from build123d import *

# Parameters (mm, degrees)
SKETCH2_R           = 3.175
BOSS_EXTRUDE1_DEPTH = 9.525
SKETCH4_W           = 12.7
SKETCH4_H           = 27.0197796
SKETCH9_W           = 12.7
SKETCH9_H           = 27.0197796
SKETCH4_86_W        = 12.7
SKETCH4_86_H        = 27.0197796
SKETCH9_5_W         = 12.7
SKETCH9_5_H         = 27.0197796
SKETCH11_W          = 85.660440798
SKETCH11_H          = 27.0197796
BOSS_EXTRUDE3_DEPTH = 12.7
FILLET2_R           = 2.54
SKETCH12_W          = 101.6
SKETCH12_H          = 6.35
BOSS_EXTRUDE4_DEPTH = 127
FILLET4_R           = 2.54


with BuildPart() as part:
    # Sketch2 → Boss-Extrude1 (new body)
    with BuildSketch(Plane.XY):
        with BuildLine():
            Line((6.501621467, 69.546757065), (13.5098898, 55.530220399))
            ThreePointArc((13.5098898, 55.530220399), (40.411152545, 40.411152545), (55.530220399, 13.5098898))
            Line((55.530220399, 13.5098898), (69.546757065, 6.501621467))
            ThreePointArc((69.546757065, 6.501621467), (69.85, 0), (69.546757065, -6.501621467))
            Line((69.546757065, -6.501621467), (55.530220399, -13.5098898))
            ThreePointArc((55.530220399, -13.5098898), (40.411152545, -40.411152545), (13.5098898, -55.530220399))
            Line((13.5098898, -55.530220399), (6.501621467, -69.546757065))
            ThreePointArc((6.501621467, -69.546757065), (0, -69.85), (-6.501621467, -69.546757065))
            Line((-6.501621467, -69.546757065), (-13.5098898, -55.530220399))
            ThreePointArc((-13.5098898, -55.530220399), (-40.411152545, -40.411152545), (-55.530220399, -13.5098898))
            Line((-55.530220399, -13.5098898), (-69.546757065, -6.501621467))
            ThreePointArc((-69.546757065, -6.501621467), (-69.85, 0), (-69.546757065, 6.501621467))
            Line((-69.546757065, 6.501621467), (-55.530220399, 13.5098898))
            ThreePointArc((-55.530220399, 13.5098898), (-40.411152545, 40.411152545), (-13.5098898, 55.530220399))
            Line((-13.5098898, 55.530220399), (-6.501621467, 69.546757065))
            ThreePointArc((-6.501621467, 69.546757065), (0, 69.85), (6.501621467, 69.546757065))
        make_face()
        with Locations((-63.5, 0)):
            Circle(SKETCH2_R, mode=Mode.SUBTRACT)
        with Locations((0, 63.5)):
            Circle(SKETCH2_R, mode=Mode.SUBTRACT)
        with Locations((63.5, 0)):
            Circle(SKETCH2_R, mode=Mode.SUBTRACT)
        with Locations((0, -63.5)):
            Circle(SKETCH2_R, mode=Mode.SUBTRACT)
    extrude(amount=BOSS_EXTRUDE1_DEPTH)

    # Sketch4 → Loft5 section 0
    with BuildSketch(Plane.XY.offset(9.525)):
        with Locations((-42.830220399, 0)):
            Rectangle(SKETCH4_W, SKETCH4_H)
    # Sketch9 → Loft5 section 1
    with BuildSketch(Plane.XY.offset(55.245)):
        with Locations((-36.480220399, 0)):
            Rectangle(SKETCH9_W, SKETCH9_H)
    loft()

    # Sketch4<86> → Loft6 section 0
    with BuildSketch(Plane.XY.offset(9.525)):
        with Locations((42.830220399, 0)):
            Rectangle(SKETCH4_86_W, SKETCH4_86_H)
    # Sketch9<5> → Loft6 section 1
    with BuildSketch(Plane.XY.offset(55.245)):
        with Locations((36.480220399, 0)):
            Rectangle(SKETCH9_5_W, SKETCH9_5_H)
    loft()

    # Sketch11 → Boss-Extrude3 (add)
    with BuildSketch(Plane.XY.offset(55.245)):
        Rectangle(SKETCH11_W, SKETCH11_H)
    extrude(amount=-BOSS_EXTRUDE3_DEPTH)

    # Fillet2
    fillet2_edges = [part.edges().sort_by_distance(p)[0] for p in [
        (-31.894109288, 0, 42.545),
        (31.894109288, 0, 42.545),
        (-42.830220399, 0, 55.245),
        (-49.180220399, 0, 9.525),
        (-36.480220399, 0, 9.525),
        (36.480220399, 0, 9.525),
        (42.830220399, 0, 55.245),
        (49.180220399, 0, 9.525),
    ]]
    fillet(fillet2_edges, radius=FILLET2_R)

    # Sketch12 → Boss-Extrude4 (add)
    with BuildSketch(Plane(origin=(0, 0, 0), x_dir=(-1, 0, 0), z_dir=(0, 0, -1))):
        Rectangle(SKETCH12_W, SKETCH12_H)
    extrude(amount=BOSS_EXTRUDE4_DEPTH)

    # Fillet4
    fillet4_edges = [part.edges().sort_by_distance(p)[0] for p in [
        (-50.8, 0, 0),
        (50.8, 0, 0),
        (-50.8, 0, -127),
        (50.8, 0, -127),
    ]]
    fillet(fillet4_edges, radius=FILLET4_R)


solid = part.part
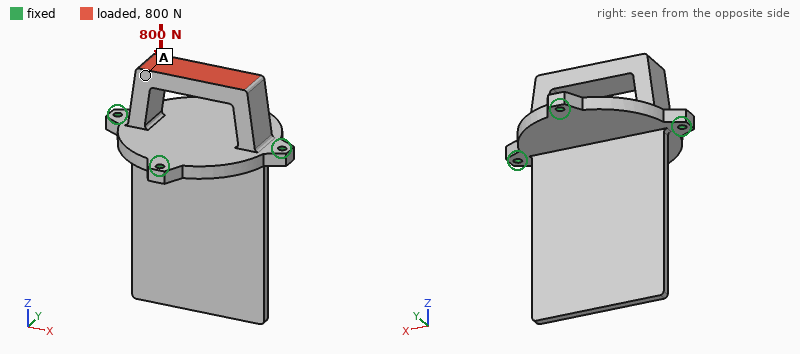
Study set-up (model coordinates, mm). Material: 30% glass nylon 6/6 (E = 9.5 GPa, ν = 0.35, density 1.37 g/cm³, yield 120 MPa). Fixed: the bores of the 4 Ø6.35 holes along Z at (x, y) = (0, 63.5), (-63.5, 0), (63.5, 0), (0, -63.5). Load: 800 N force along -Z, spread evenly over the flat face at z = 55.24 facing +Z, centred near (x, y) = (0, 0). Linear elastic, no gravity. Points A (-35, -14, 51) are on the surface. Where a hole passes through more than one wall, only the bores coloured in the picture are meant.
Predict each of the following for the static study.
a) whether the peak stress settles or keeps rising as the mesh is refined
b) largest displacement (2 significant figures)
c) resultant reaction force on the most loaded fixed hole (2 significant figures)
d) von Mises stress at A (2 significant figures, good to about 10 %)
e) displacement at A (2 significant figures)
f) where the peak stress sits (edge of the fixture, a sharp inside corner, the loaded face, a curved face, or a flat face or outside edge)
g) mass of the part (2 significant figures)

keeps rising
54 µm
380 N
1.3 MPa
22 µm
edge of the fixture
330 g
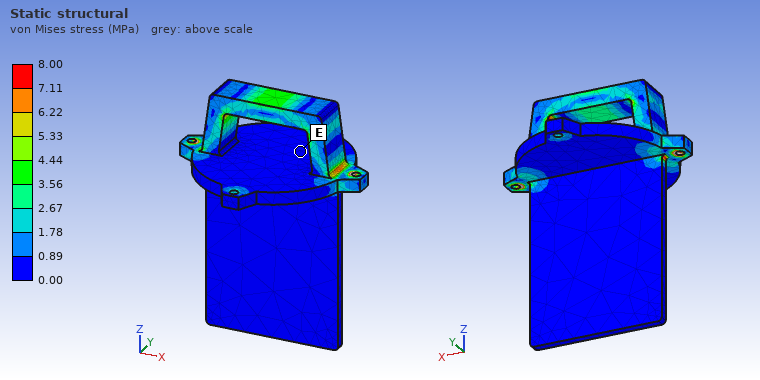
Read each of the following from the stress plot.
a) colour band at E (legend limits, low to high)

0.00 to 0.89 MPa
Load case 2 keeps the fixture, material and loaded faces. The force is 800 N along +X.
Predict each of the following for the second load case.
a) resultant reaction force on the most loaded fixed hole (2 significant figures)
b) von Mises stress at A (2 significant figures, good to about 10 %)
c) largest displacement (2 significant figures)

490 N
3.5 MPa
0.11 mm
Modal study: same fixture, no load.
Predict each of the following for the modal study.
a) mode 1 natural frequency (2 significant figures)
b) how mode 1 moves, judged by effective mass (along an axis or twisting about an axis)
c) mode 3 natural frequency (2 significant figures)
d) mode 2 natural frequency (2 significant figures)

160 Hz
along Y
980 Hz
470 Hz
